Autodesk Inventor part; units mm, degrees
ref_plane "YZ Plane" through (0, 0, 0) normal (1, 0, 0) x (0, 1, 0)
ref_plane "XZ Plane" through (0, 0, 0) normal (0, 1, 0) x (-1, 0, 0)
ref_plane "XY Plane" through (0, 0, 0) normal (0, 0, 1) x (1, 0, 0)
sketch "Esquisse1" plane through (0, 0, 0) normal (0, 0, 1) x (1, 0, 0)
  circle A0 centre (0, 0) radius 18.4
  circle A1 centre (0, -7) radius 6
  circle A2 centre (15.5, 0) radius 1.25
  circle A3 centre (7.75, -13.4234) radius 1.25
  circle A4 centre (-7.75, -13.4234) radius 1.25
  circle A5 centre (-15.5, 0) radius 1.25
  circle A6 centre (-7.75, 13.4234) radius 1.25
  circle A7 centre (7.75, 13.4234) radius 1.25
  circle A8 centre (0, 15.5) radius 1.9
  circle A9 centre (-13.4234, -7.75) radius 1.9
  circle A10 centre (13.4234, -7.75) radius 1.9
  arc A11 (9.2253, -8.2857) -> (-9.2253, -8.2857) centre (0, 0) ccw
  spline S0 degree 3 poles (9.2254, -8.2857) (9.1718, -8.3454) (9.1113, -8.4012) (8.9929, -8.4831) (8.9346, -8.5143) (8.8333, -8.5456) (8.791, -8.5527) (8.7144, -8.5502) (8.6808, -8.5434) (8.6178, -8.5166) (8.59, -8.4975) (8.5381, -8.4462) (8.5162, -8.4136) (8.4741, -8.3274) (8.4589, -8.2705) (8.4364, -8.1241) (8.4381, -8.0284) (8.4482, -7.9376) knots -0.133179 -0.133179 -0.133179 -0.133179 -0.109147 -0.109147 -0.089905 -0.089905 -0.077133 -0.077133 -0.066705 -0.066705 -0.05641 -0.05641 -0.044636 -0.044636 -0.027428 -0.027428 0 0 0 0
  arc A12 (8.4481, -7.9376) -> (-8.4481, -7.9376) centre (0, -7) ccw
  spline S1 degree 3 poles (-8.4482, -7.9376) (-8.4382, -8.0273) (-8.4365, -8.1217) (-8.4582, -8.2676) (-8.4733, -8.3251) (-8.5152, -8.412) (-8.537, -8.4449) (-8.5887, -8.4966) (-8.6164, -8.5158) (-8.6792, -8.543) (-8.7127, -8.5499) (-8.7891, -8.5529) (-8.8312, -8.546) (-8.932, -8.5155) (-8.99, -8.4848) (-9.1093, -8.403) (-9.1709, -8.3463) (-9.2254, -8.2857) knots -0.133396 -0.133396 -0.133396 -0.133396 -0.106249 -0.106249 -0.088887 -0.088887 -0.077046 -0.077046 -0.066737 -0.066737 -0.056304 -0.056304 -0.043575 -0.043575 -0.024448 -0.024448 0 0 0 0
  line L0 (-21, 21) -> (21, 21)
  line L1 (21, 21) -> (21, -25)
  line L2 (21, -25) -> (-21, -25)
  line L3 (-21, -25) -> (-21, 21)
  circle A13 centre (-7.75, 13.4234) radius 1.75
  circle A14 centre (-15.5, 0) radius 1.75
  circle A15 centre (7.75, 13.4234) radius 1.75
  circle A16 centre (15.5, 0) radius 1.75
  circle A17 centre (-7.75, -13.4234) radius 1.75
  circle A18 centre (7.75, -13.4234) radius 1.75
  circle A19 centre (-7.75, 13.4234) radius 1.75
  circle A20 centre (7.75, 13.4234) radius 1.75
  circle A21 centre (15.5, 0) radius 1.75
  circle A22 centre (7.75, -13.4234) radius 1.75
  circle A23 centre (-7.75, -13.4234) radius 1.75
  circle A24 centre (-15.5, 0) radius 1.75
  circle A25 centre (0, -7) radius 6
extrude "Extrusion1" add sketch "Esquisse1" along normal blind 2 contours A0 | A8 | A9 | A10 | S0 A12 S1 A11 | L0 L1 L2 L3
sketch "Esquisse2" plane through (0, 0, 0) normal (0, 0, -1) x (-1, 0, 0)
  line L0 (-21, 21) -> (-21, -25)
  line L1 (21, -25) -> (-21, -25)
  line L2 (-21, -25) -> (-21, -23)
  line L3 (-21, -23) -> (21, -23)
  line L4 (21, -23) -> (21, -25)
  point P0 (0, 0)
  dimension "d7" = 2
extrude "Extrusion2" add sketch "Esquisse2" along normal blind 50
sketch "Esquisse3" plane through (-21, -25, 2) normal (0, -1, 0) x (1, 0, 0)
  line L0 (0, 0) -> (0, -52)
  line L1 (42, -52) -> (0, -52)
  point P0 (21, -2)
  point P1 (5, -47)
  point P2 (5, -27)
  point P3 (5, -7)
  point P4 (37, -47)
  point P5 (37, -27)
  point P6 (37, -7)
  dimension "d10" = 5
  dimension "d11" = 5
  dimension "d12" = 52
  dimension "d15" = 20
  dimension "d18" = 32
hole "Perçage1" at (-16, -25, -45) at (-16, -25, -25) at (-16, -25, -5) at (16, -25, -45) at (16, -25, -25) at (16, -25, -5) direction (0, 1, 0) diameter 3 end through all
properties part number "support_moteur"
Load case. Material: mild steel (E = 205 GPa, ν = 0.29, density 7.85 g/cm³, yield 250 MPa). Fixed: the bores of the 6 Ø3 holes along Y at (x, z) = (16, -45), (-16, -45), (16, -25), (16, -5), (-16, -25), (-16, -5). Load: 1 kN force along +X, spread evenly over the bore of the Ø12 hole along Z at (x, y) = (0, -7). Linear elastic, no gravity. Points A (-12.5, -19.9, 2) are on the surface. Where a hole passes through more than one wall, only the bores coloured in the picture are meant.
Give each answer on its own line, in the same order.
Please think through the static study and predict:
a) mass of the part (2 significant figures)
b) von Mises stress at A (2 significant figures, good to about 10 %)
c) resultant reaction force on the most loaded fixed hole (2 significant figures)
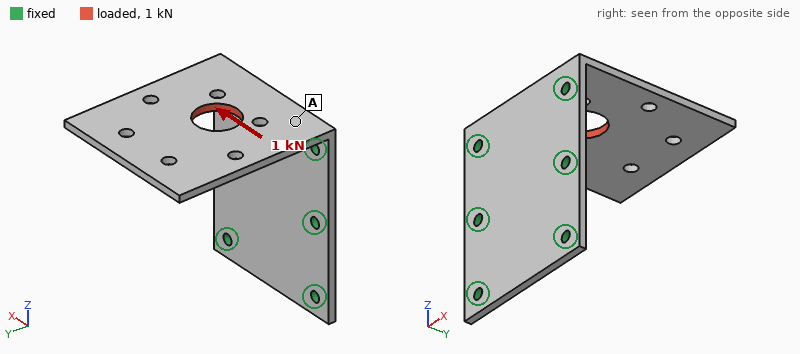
60 g
19 MPa
720 N
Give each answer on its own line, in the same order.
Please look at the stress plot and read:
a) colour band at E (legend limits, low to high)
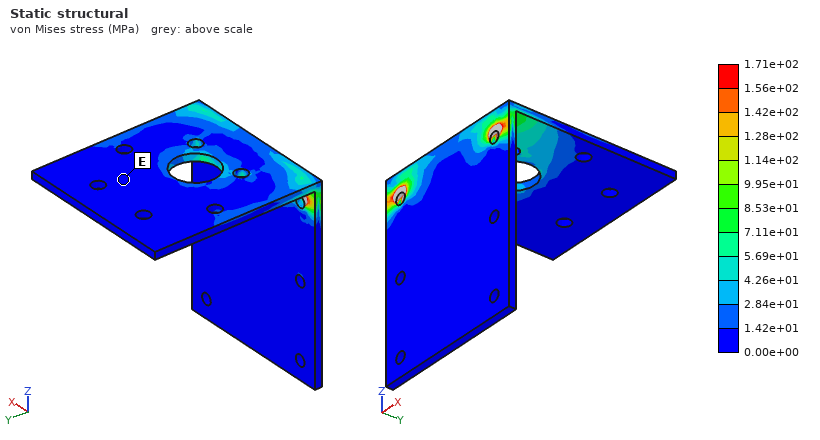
0.00e+00 to 1.42e+01 MPa
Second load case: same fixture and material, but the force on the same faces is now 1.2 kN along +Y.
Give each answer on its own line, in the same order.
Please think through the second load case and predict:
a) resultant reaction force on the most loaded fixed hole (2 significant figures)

650 N
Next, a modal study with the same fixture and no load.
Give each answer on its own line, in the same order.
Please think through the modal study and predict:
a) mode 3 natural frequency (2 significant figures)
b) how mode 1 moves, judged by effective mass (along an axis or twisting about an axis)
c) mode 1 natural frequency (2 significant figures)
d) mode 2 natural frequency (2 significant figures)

4200 Hz
along Z
650 Hz
1800 Hz
